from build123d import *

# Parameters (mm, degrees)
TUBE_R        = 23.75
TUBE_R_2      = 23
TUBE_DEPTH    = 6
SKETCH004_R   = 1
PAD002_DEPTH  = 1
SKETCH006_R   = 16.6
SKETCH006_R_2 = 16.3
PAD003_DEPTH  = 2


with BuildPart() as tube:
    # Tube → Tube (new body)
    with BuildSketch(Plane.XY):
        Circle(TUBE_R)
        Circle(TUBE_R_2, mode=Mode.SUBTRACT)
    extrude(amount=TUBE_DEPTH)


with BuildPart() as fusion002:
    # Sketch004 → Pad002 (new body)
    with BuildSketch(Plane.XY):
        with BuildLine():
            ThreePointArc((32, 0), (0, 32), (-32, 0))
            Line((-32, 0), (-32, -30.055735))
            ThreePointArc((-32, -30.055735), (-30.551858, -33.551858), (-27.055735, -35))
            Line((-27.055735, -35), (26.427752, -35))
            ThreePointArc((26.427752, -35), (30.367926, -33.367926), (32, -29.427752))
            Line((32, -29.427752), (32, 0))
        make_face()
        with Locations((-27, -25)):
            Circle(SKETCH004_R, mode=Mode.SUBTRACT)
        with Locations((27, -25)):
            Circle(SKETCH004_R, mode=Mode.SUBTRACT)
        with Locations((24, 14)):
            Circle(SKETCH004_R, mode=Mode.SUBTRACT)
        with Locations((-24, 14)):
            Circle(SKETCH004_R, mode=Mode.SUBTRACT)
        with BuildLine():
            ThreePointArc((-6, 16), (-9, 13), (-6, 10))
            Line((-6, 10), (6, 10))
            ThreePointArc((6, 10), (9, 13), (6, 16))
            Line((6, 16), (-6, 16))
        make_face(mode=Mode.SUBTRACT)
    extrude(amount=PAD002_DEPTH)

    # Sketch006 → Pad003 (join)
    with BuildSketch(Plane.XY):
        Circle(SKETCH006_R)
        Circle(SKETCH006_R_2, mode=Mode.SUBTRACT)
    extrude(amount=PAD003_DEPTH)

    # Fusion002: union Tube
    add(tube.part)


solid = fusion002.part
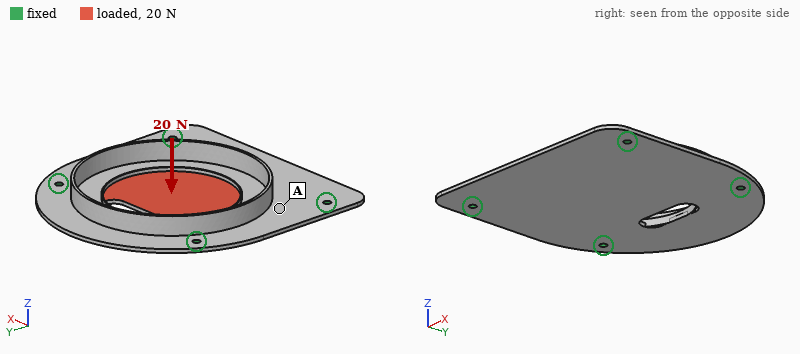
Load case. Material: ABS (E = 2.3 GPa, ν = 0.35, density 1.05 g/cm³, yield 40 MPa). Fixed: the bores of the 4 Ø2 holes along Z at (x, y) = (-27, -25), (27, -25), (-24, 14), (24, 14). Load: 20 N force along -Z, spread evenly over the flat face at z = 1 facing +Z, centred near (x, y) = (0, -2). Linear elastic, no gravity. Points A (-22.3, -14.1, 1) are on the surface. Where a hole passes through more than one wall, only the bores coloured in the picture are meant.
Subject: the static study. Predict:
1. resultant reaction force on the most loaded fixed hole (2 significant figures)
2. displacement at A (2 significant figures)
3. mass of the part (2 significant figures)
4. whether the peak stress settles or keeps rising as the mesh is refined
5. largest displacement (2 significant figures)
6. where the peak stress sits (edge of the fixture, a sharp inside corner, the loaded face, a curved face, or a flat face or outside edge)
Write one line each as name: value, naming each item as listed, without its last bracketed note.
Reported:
resultant reaction force on the most loaded fixed hole: 6.8 N
displacement at A: 0.24 mm
mass of the part: 4.5 g
whether the peak stress settles or keeps rising as the mesh is refined: keeps rising
largest displacement: 1.0 mm
where the peak stress sits: edge of the fixture
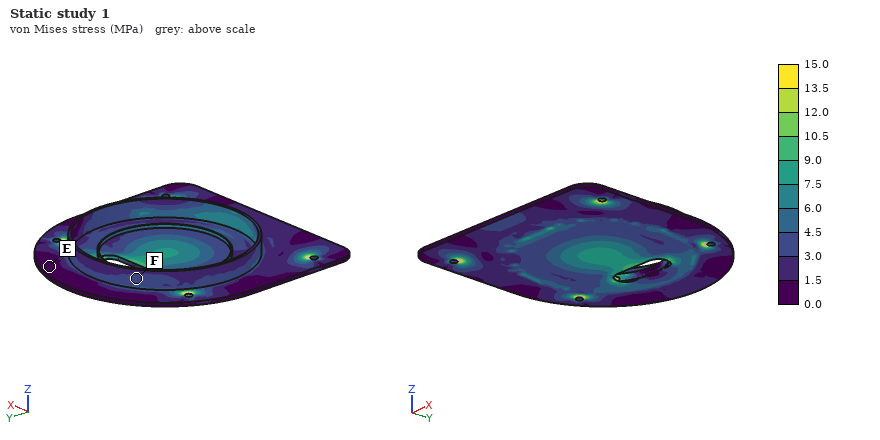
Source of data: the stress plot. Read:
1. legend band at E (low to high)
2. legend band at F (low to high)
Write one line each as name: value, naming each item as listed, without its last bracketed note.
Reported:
legend band at E: 0.0 to 1.5 MPa
legend band at F: 3.0 to 4.5 MPa
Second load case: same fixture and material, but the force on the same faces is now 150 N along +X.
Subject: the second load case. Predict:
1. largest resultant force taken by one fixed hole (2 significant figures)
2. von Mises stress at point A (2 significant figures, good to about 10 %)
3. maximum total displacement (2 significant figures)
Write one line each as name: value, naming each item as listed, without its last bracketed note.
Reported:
largest resultant force taken by one fixed hole: 42 N
von Mises stress at point A: 2.3 MPa
maximum total displacement: 78 µm
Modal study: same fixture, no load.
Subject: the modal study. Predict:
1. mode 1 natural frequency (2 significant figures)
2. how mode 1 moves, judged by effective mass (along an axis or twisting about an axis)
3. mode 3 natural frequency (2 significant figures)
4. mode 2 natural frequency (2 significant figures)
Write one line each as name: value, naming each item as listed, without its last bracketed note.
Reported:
mode 1 natural frequency: 570 Hz
how mode 1 moves, judged by effective mass: along Z
mode 3 natural frequency: 960 Hz
mode 2 natural frequency: 700 Hz
